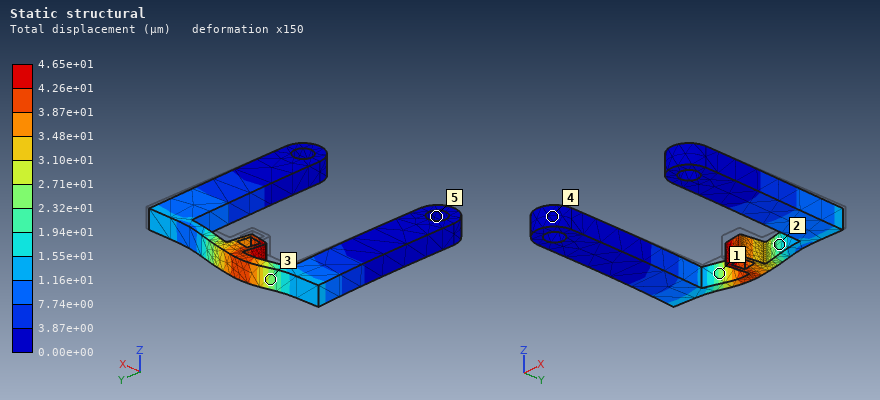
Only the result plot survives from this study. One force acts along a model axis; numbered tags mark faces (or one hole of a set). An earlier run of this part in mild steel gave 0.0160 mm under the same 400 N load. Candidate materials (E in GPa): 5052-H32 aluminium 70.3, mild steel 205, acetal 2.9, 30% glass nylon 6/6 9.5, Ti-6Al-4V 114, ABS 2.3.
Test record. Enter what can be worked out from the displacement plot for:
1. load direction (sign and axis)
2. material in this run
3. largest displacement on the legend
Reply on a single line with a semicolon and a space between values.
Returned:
+Y; 5052-H32 aluminium; 4.65e+01 µm
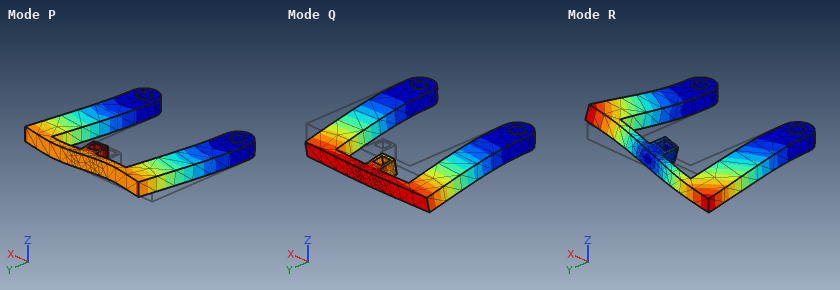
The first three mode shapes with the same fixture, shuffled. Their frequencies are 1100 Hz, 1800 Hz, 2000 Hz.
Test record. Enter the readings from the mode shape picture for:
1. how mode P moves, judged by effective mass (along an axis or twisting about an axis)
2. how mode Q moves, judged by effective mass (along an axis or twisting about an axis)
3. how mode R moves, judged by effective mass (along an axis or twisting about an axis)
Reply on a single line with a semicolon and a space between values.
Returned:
along X; along Z; twisting about Y
